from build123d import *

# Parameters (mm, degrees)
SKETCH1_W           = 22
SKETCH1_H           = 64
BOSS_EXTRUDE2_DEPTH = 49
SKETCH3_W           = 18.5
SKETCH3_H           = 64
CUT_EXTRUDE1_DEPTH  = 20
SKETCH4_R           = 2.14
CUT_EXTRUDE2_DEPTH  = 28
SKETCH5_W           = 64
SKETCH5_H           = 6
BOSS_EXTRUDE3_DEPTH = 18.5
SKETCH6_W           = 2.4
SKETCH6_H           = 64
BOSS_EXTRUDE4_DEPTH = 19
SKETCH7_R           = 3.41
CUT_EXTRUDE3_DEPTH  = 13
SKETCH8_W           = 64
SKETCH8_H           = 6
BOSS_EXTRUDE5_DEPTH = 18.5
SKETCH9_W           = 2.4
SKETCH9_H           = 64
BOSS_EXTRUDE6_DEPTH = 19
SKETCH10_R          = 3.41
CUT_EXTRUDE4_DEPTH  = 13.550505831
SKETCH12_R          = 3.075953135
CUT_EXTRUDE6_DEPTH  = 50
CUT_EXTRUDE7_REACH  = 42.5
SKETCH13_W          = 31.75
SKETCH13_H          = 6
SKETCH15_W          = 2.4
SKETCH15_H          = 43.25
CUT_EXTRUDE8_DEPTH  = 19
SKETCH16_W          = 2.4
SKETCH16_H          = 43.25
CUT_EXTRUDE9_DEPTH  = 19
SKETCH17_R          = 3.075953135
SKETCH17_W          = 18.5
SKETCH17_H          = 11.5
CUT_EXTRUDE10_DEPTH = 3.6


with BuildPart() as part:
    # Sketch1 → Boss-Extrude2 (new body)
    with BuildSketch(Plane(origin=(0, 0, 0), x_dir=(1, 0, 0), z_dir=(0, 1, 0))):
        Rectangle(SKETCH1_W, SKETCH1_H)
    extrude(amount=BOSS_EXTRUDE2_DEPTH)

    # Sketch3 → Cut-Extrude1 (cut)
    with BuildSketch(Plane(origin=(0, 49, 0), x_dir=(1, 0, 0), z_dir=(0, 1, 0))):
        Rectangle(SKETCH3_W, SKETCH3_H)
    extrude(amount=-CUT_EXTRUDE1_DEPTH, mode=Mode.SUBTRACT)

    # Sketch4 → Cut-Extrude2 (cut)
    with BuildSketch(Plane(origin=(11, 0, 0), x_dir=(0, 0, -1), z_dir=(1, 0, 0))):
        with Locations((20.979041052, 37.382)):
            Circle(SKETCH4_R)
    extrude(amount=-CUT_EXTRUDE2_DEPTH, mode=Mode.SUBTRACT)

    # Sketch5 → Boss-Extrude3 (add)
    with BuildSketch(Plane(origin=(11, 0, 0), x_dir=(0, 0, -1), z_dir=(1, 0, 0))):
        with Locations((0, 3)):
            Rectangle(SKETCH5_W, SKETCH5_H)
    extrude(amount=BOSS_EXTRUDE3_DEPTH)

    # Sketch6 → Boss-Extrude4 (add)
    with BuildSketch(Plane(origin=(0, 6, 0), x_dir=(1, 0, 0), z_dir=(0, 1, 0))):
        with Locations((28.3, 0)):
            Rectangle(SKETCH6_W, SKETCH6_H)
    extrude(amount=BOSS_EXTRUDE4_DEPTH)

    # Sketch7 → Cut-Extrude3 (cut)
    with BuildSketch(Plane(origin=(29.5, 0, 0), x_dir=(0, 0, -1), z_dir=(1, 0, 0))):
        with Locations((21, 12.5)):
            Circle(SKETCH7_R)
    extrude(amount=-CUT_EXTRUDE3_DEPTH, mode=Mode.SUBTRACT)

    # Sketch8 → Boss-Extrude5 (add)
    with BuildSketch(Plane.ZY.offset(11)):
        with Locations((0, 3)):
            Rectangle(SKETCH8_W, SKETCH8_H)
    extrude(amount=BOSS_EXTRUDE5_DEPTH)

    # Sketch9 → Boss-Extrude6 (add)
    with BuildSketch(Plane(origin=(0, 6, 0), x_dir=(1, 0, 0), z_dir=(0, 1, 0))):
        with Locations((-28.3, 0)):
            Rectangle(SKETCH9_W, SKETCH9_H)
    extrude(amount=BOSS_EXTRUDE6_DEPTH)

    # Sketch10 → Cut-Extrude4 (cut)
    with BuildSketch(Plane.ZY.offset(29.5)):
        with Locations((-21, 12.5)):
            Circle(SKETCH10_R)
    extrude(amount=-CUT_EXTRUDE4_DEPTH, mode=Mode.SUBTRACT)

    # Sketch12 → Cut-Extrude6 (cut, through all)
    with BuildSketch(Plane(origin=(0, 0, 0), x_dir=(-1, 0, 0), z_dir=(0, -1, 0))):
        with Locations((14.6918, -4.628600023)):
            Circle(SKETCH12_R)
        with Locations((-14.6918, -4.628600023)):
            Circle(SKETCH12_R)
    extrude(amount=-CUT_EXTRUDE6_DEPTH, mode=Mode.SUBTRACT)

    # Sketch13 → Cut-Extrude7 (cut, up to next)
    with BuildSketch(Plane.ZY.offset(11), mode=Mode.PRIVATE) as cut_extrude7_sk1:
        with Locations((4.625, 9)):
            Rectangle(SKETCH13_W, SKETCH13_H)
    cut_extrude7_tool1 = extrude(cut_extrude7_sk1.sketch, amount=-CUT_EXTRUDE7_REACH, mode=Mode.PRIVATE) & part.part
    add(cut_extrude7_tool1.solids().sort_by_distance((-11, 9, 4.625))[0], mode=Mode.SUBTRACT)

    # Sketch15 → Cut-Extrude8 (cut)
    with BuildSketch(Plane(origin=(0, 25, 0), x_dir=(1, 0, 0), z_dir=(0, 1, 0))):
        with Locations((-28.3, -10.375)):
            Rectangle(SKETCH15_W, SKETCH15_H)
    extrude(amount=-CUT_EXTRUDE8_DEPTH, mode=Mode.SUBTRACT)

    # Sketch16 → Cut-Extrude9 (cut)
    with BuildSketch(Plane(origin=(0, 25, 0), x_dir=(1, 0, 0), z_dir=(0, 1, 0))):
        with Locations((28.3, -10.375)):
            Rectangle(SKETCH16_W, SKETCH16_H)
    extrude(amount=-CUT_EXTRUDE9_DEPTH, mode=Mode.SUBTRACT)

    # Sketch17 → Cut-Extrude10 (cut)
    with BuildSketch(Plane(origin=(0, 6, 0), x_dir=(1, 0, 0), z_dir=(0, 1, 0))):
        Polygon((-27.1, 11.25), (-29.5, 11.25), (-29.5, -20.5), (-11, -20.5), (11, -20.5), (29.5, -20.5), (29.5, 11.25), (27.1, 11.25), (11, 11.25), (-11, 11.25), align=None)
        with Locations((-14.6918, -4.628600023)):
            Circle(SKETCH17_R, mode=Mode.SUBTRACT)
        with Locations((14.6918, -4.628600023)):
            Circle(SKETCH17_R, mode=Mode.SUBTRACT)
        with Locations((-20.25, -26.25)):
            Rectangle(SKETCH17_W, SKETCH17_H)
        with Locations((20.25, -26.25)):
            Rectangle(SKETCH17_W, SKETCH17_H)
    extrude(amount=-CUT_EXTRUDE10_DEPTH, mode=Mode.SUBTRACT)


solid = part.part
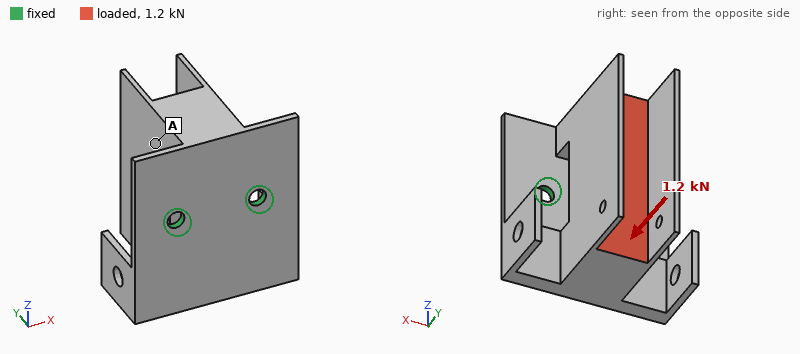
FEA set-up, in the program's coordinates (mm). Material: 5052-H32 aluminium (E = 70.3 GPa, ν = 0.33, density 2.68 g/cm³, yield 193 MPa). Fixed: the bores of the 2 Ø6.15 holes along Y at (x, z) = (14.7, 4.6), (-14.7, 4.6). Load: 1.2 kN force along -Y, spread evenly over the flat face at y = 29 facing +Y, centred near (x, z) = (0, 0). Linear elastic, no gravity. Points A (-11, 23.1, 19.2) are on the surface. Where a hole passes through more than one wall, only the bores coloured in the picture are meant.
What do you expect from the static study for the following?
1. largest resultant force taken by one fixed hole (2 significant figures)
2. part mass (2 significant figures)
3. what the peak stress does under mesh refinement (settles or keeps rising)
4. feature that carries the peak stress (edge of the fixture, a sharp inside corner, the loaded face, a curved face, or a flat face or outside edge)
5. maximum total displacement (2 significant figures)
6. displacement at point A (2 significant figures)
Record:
610 N
130 g
keeps rising
edge of the fixture
0.18 mm
0.056 mm
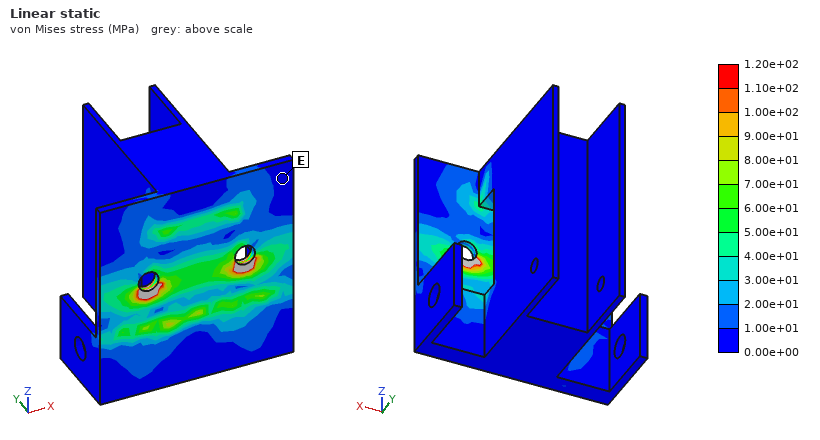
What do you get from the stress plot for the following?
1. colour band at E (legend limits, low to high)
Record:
0.00e+00 to 1.00e+01 MPa
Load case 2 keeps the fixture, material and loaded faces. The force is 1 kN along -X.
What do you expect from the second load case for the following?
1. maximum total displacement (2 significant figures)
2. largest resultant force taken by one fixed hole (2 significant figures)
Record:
0.31 mm
990 N
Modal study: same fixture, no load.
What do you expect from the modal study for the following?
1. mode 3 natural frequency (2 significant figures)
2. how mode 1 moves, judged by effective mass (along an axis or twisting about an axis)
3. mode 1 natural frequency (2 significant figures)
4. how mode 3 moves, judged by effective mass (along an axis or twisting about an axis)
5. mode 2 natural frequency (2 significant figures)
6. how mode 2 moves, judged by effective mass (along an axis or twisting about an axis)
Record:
2200 Hz
along Z
700 Hz
along Y
1400 Hz
along X
